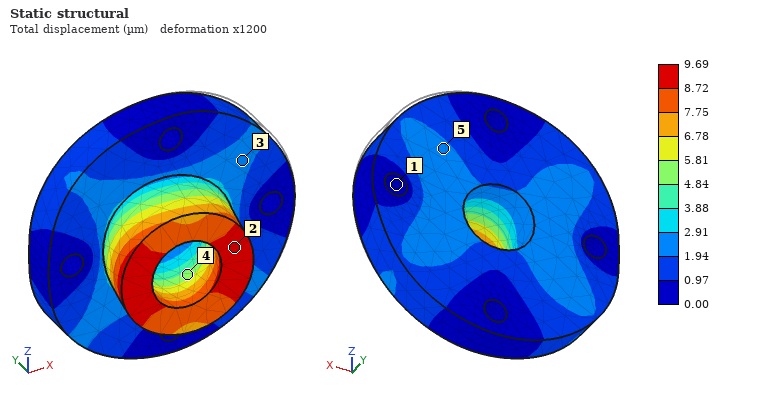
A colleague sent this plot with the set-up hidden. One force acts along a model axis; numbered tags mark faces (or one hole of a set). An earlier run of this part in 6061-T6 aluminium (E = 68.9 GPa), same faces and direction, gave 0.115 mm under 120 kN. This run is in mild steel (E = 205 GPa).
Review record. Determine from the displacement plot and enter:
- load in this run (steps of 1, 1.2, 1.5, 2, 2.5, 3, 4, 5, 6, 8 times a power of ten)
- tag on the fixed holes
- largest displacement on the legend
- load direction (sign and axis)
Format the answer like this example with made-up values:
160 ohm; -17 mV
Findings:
30 kN; 1; 9.69 µm; -X
